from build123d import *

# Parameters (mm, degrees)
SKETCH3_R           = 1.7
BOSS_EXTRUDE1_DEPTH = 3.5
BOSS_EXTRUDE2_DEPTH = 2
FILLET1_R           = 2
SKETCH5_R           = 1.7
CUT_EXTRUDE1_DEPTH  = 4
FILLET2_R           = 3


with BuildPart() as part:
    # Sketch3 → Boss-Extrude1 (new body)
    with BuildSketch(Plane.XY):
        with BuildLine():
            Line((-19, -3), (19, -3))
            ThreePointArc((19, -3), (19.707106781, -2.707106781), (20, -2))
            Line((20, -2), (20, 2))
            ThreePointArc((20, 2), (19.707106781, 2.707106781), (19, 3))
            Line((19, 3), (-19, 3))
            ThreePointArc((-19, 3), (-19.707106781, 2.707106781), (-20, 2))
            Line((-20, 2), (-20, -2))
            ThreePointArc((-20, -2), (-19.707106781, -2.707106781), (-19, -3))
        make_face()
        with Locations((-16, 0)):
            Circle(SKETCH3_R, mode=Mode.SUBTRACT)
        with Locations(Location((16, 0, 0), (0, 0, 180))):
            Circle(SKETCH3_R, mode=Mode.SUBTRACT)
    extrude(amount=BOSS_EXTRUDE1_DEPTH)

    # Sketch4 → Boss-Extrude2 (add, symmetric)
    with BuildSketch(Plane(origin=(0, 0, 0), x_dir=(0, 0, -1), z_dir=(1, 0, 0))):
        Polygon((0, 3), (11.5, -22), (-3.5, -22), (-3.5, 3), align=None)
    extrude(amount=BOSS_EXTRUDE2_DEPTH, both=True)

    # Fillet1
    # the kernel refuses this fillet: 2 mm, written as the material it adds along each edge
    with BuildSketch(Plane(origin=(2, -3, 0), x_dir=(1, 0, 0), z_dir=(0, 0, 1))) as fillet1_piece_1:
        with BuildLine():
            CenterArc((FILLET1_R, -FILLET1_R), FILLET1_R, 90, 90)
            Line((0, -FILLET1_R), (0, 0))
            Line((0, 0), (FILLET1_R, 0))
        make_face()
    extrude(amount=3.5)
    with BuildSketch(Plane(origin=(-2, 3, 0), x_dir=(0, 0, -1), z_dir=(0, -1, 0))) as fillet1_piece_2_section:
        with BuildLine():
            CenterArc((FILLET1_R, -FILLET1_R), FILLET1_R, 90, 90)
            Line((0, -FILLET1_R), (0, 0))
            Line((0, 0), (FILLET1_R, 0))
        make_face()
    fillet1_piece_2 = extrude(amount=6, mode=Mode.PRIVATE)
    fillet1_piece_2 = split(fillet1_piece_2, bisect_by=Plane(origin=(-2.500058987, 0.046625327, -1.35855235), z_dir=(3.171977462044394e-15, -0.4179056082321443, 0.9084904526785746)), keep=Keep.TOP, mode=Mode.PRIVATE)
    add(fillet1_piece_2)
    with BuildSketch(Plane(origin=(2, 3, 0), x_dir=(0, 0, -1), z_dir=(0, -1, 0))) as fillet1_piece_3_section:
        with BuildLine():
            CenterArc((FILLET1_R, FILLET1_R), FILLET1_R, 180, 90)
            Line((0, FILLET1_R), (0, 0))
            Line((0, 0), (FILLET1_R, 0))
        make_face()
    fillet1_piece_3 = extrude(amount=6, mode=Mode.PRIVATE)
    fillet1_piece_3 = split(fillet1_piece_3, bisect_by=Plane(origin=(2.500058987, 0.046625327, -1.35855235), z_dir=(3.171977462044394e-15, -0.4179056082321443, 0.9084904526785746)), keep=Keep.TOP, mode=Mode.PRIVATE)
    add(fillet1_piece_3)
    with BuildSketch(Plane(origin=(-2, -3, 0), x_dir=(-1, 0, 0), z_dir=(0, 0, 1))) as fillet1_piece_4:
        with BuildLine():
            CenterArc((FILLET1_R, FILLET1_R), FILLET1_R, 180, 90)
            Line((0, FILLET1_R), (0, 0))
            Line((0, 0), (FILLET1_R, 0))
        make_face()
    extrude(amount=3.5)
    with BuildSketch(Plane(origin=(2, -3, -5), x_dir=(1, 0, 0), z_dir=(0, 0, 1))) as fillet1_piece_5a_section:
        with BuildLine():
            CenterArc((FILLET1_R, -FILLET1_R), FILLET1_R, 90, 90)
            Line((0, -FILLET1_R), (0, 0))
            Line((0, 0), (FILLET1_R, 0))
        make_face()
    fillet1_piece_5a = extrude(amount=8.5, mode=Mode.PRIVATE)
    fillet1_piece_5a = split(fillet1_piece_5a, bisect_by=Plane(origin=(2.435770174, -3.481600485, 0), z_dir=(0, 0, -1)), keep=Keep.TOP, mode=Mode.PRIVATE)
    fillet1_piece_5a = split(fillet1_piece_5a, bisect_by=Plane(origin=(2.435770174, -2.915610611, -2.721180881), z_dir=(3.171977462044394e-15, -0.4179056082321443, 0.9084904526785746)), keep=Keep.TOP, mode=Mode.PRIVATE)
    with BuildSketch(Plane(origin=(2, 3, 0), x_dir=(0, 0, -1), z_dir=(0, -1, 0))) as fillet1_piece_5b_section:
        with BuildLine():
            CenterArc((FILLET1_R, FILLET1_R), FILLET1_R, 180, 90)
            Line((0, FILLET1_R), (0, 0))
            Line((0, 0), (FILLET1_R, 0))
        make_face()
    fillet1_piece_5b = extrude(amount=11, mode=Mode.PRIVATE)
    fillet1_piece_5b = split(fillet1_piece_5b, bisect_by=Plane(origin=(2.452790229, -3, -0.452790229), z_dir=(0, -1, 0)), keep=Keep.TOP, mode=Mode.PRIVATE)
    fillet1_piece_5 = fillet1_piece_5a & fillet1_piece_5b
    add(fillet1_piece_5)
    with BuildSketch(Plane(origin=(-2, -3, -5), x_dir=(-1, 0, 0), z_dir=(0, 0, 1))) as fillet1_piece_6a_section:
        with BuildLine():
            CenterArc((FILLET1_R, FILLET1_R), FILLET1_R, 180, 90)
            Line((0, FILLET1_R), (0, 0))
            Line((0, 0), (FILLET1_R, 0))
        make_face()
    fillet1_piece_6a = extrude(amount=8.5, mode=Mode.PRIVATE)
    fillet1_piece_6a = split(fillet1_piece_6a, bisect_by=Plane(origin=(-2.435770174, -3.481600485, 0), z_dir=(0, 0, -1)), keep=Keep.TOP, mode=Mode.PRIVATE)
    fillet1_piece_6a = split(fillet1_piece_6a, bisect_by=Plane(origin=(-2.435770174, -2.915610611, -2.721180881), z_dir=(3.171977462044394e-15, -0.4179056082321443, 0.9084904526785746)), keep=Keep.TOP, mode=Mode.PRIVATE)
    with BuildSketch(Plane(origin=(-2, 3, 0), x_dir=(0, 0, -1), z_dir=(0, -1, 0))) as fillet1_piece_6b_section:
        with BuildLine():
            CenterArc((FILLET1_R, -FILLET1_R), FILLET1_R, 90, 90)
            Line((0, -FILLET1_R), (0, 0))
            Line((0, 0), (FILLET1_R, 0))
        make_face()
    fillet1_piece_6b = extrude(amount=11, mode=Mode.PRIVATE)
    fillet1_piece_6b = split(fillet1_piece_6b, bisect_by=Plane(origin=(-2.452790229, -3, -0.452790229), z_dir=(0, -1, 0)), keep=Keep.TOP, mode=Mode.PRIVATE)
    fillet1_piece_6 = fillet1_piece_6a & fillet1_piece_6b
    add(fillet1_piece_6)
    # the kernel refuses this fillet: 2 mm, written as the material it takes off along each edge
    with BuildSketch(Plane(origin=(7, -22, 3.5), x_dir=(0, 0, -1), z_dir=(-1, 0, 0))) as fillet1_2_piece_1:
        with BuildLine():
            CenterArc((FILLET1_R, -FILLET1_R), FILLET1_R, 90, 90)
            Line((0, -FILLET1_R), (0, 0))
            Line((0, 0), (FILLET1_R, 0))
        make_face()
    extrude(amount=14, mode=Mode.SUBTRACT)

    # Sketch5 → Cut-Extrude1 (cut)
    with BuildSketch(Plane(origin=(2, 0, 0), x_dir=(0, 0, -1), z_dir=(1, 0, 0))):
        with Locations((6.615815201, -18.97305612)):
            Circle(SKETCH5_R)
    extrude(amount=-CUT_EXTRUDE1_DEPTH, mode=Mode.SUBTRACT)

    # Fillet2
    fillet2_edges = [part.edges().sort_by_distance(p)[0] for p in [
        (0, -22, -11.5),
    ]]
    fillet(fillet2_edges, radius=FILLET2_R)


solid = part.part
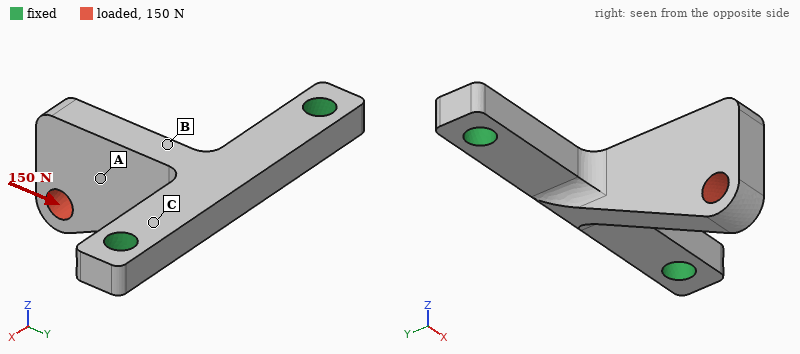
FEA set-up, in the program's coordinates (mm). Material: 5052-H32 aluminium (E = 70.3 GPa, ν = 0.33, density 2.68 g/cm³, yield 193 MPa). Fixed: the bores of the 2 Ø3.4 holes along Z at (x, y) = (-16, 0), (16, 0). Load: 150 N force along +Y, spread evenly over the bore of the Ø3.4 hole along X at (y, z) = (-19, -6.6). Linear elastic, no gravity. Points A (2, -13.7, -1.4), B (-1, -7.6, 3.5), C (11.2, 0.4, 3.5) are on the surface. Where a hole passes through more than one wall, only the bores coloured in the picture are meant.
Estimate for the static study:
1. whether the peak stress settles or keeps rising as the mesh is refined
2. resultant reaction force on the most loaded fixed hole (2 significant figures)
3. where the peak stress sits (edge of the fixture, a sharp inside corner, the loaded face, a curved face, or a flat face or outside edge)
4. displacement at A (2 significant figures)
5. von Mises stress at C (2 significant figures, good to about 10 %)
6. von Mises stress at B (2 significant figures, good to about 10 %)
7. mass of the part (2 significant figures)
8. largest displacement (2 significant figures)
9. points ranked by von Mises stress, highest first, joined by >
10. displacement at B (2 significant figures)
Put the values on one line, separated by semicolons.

keeps rising; 75 N; edge of the fixture; 0.092 mm; 46 MPa; 17 MPa; 4.2 g; 0.16 mm; C > B > A; 0.047 mm
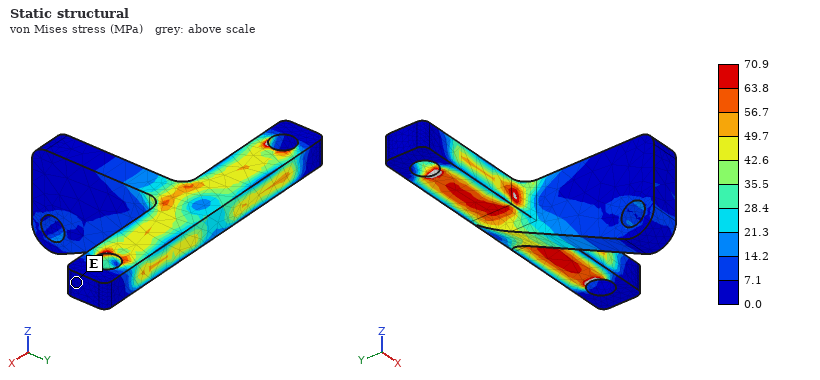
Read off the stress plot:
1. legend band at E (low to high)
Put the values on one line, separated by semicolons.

0.0 to 7.1 MPa
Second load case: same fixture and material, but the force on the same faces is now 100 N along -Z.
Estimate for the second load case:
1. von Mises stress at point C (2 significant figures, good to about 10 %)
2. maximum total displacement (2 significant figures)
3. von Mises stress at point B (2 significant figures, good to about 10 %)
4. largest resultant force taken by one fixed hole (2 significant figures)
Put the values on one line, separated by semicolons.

85 MPa; 0.24 mm; 29 MPa; 55 N
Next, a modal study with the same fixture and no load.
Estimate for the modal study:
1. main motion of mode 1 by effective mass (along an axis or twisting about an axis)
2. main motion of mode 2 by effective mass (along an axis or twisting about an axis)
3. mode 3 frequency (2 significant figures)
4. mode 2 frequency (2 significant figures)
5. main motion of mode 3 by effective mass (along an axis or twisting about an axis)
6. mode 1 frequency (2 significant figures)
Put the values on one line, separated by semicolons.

along Z; along X; 14 kHz; 5800 Hz; along Y; 3200 Hz
